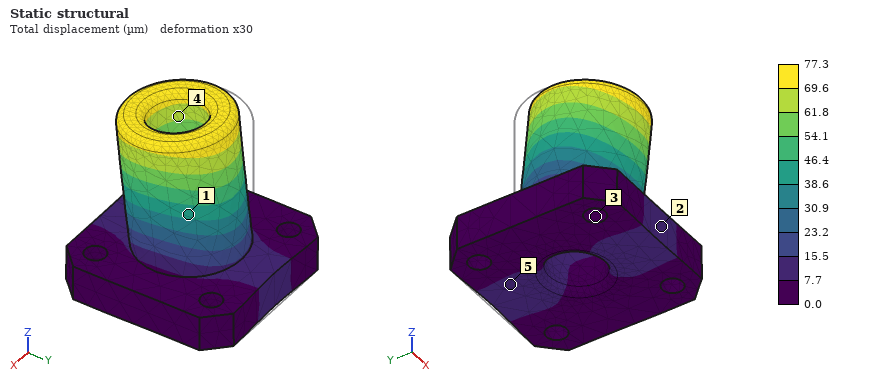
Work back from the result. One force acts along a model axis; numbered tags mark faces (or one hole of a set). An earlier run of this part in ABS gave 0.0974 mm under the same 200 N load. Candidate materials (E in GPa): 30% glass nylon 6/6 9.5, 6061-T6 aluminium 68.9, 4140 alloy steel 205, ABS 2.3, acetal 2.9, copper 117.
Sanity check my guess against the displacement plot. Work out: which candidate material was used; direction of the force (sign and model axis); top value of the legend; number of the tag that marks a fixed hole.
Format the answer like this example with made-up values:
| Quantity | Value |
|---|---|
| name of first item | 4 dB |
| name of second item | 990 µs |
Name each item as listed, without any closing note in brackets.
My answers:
| Quantity | Value |
|---|---|
| which candidate material was used | acetal |
| direction of the force | -Y |
| top value of the legend | 77.3 µm |
| number of the tag that marks a fixed hole | 3 |
